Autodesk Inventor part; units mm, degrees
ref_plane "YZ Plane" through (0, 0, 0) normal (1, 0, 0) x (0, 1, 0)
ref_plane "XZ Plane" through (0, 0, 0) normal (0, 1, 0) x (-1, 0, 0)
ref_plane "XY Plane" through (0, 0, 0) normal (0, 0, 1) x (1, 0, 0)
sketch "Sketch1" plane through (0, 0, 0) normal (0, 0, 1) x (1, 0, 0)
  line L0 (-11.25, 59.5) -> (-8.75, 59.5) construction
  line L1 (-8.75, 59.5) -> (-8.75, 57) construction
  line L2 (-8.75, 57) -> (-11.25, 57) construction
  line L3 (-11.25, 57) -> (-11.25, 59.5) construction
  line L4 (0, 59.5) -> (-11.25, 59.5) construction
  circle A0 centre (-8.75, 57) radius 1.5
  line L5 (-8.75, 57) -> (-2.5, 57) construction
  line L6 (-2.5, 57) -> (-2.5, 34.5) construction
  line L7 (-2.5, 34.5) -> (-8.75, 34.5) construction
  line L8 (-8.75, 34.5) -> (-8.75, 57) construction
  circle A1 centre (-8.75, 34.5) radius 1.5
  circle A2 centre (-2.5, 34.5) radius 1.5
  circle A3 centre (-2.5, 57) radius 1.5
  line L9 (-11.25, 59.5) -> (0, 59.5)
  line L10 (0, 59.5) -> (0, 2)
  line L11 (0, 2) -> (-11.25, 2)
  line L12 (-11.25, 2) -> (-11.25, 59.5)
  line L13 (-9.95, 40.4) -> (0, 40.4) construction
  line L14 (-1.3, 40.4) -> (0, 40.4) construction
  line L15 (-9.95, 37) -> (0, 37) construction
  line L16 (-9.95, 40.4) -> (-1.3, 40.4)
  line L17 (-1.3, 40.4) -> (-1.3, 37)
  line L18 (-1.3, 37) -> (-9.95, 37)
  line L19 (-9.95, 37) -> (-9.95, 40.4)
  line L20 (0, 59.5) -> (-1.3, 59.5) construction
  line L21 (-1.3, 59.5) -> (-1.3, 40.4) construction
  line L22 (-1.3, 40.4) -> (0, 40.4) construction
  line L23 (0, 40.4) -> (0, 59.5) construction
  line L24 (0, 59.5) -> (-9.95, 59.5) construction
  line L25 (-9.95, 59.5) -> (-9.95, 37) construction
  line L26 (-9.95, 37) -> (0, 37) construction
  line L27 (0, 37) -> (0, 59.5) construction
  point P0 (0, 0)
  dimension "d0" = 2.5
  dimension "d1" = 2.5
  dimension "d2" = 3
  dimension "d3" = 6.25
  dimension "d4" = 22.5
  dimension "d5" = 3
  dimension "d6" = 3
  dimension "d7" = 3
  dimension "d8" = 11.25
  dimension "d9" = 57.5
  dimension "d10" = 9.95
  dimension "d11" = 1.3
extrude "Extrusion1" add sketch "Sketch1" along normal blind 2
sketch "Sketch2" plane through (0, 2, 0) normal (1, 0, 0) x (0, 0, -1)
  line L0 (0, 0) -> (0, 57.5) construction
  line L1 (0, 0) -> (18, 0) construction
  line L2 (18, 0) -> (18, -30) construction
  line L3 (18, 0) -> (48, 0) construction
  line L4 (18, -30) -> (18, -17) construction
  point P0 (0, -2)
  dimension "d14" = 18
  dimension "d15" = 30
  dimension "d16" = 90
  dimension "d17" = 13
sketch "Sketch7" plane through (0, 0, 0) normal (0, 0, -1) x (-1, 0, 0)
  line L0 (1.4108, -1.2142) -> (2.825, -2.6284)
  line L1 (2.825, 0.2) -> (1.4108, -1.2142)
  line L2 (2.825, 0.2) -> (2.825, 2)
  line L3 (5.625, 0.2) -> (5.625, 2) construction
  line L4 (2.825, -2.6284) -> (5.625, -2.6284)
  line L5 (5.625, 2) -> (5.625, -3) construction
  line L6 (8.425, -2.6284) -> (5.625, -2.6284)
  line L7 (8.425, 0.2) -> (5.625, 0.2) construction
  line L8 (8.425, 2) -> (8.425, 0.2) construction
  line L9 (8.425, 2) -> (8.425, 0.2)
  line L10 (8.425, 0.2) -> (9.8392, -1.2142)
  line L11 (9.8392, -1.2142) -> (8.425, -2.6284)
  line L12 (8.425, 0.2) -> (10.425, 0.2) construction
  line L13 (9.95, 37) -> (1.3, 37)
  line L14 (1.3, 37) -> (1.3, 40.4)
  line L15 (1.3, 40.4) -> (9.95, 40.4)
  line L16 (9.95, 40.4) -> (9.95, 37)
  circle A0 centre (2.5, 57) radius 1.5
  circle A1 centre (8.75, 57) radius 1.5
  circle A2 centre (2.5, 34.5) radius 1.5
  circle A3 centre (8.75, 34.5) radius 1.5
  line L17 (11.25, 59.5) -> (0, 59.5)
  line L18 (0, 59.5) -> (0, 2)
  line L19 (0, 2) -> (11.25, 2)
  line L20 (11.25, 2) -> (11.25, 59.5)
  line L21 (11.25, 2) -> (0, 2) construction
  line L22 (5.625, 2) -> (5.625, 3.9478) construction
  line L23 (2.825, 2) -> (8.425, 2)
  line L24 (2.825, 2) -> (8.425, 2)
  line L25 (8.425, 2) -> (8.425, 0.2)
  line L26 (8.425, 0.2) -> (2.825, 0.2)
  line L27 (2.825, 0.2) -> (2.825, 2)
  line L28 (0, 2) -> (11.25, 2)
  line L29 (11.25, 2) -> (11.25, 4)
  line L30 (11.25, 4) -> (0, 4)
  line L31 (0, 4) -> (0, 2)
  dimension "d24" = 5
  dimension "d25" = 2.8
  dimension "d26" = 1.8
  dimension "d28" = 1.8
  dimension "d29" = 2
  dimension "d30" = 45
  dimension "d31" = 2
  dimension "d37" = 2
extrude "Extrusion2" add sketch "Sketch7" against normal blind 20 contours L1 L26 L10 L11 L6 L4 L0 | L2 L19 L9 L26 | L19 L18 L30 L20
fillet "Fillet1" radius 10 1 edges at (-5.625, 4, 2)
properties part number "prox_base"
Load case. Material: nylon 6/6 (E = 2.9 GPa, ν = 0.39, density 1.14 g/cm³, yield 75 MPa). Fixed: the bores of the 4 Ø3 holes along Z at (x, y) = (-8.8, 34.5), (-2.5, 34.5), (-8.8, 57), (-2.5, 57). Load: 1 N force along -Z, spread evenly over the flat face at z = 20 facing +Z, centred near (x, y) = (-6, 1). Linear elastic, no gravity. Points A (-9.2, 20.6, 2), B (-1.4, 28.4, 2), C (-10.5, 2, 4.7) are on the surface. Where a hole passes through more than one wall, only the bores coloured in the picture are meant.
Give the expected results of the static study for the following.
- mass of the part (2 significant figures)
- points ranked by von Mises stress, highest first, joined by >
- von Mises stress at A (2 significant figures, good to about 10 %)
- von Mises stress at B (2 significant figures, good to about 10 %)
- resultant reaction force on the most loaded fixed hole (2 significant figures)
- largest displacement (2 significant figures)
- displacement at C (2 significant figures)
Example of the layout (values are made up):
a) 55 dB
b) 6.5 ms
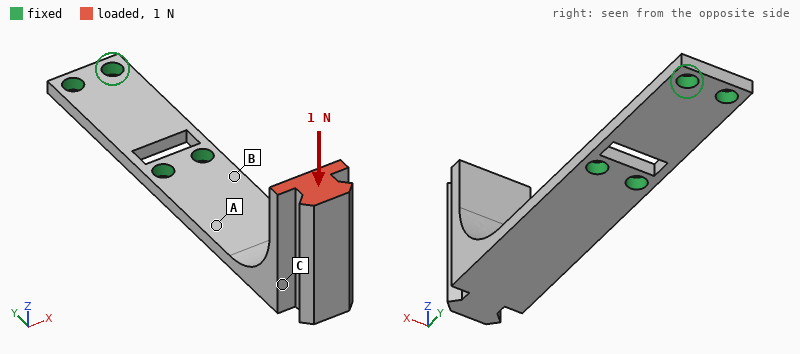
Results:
a) 2.8 g
b) B > A > C
c) 2.6 MPa
d) 3.6 MPa
e) 0.50 N
f) 0.70 mm
g) 0.48 mm
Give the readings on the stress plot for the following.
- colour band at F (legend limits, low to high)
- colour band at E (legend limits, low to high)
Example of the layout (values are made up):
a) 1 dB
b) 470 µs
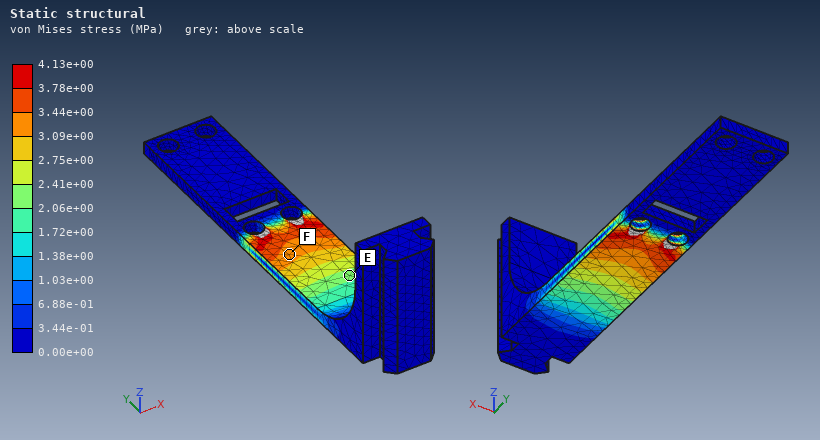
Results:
a) 3.09e+00 to 3.44e+00 MPa
b) 2.06e+00 to 2.41e+00 MPa
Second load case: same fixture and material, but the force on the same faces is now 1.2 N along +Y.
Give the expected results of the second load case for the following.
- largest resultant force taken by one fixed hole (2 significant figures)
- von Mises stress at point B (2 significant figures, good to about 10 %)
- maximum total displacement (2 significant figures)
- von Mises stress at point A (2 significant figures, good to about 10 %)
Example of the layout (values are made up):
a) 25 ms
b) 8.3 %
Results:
a) 0.61 N
b) 3.1 MPa
c) 0.73 mm
d) 3.1 MPa
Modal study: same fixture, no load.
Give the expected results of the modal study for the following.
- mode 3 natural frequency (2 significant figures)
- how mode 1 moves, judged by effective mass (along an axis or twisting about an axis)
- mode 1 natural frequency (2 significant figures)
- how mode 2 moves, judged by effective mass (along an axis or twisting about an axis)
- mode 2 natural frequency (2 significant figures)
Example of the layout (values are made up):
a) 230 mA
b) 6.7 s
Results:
a) 1100 Hz
b) along Z
c) 170 Hz
d) along X
e) 460 Hz
